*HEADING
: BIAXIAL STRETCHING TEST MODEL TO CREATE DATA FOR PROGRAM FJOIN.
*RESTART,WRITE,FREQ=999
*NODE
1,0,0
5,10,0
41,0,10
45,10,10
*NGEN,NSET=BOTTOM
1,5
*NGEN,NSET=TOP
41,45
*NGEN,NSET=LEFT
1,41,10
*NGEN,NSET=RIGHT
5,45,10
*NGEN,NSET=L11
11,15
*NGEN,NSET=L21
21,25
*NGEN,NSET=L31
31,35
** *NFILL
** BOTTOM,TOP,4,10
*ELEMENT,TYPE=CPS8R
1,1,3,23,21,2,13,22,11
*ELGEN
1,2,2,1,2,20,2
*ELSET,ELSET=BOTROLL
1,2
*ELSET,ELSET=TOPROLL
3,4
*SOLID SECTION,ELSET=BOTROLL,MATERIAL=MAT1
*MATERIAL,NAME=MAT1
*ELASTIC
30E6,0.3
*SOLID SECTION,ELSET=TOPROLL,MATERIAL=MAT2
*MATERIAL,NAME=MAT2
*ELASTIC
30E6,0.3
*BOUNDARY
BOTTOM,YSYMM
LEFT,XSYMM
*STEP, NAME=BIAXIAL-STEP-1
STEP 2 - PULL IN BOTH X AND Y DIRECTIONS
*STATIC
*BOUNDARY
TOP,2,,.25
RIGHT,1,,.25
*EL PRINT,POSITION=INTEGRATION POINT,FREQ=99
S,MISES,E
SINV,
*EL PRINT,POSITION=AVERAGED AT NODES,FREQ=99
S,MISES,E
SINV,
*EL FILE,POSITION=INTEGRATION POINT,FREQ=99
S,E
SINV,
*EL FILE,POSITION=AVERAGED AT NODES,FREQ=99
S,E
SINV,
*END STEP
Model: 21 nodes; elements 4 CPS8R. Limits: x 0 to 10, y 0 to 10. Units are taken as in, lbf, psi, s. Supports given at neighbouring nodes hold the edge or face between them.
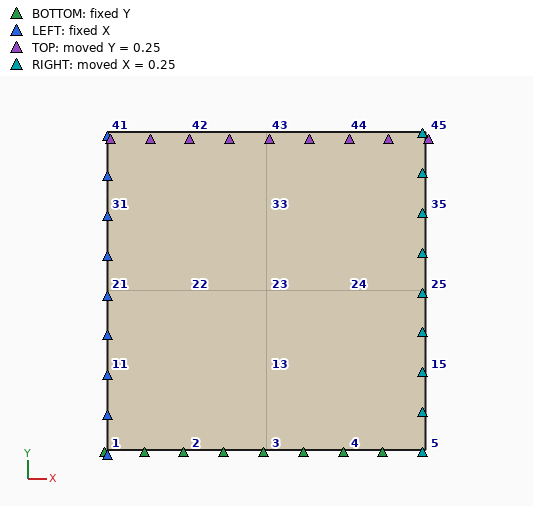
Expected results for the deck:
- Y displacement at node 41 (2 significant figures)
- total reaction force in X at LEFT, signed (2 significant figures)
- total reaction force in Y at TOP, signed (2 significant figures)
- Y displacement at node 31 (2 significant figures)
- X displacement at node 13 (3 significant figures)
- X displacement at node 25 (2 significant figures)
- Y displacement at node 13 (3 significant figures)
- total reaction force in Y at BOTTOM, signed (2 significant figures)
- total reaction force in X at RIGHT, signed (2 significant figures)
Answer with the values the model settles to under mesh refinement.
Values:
0.25 in
-1.1e+07 lbf
1.1e+07 lbf
0.19 in
0.125 in
0.25 in
0.0625 in
-1.1e+07 lbf
1.1e+07 lbf
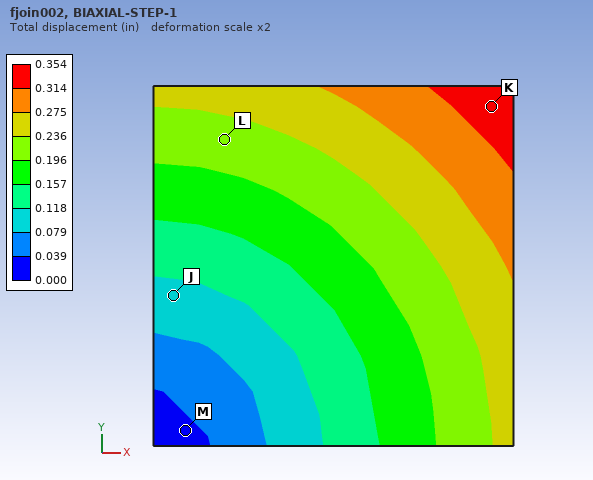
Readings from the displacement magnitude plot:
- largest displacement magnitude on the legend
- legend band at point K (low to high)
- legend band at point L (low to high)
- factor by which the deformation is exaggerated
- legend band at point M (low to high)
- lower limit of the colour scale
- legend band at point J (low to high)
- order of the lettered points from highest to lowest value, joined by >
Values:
0.354 in
0.314 to 0.354 in
0.196 to 0.236 in
2
0.000 to 0.039 in
0.000 in
0.079 to 0.118 in
K > L > J > M
